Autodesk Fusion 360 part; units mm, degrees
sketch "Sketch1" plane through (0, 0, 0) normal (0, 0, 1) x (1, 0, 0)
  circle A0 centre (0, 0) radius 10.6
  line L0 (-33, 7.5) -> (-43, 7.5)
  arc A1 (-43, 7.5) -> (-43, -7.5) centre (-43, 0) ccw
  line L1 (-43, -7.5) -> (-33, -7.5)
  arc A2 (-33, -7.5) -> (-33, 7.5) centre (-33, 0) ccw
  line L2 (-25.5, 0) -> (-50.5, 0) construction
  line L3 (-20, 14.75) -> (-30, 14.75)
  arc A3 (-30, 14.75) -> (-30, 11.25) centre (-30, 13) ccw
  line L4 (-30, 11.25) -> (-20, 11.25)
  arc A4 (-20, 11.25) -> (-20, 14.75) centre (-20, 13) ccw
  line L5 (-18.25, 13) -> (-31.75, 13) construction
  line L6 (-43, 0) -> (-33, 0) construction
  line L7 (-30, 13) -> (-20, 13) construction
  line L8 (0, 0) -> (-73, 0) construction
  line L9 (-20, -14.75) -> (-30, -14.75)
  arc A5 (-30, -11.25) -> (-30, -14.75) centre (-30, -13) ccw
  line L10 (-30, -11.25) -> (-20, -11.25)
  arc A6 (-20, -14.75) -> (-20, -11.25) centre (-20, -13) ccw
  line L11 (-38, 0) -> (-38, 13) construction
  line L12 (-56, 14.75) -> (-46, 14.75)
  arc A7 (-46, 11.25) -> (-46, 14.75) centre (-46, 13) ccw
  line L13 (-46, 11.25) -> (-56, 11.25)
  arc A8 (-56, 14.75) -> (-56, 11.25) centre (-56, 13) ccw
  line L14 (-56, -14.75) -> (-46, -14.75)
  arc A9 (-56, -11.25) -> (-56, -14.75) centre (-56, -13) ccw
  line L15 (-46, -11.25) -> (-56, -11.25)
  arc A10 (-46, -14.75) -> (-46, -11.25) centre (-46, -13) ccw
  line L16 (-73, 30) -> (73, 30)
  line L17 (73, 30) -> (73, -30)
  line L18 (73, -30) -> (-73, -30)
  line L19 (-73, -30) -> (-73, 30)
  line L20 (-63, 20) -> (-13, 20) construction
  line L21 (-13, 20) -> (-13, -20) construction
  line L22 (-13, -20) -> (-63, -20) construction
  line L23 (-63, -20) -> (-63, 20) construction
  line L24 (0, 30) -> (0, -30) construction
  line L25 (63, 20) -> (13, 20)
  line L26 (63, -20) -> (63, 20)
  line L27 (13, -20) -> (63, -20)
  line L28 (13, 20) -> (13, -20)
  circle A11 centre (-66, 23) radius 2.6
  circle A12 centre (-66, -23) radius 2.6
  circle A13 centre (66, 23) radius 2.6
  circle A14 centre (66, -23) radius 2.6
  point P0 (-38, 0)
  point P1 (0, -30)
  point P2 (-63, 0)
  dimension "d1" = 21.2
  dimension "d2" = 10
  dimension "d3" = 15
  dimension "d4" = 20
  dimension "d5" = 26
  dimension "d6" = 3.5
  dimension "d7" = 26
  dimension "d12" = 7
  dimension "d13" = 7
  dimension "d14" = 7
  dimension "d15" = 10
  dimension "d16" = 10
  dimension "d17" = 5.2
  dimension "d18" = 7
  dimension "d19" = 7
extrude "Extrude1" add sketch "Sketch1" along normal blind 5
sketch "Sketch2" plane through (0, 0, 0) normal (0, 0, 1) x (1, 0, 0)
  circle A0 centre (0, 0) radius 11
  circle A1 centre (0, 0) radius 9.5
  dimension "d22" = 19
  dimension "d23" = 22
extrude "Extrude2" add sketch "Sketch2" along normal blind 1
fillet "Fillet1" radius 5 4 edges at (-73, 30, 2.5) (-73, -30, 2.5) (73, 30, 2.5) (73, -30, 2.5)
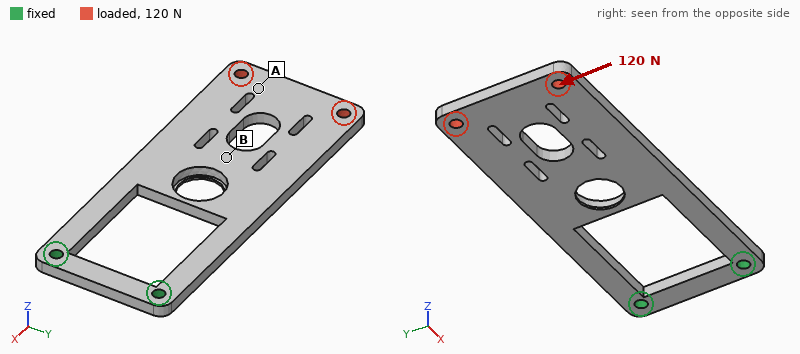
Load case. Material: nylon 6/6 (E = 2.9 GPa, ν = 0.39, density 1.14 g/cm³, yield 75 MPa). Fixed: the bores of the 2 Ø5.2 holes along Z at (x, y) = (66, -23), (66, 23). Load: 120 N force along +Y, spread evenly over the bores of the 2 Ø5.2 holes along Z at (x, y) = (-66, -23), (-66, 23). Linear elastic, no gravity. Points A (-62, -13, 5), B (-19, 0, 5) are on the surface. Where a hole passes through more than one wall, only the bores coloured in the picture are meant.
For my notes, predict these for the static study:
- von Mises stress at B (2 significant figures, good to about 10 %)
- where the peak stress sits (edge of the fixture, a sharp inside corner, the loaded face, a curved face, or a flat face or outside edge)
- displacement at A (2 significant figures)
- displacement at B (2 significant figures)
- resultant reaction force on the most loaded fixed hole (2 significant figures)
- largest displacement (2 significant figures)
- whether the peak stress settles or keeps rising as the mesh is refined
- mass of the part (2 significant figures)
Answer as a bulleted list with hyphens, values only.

- 4.1 MPa
- edge of the fixture
- 1.6 mm
- 1.3 mm
- 260 N
- 1.6 mm
- keeps rising
- 33 g
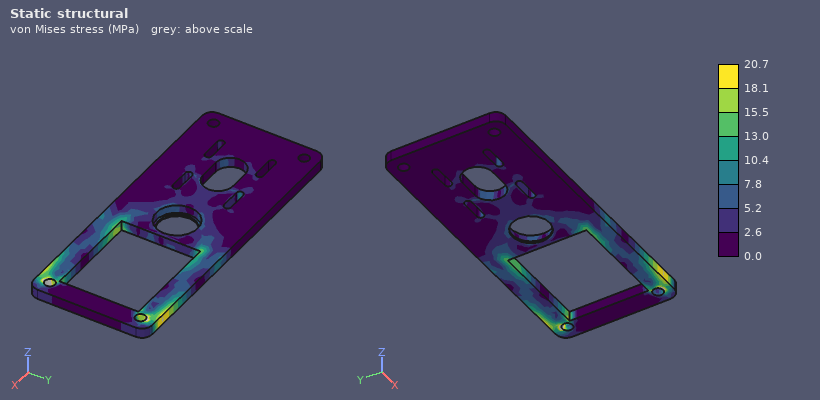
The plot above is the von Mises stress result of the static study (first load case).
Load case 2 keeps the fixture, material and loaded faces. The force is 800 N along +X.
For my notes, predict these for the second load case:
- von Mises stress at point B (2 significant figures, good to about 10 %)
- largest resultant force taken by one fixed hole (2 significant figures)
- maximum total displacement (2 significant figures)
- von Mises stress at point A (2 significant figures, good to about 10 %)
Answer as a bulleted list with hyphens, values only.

- 1.1 MPa
- 400 N
- 0.29 mm
- 2.6 MPa
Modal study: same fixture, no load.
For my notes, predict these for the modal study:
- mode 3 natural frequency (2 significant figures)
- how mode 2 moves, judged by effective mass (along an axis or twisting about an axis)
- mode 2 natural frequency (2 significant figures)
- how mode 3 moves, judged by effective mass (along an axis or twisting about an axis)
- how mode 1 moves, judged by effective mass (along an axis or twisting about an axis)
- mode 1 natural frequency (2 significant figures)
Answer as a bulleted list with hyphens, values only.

- 310 Hz
- twisting about X
- 220 Hz
- along Y
- along Z
- 44 Hz
